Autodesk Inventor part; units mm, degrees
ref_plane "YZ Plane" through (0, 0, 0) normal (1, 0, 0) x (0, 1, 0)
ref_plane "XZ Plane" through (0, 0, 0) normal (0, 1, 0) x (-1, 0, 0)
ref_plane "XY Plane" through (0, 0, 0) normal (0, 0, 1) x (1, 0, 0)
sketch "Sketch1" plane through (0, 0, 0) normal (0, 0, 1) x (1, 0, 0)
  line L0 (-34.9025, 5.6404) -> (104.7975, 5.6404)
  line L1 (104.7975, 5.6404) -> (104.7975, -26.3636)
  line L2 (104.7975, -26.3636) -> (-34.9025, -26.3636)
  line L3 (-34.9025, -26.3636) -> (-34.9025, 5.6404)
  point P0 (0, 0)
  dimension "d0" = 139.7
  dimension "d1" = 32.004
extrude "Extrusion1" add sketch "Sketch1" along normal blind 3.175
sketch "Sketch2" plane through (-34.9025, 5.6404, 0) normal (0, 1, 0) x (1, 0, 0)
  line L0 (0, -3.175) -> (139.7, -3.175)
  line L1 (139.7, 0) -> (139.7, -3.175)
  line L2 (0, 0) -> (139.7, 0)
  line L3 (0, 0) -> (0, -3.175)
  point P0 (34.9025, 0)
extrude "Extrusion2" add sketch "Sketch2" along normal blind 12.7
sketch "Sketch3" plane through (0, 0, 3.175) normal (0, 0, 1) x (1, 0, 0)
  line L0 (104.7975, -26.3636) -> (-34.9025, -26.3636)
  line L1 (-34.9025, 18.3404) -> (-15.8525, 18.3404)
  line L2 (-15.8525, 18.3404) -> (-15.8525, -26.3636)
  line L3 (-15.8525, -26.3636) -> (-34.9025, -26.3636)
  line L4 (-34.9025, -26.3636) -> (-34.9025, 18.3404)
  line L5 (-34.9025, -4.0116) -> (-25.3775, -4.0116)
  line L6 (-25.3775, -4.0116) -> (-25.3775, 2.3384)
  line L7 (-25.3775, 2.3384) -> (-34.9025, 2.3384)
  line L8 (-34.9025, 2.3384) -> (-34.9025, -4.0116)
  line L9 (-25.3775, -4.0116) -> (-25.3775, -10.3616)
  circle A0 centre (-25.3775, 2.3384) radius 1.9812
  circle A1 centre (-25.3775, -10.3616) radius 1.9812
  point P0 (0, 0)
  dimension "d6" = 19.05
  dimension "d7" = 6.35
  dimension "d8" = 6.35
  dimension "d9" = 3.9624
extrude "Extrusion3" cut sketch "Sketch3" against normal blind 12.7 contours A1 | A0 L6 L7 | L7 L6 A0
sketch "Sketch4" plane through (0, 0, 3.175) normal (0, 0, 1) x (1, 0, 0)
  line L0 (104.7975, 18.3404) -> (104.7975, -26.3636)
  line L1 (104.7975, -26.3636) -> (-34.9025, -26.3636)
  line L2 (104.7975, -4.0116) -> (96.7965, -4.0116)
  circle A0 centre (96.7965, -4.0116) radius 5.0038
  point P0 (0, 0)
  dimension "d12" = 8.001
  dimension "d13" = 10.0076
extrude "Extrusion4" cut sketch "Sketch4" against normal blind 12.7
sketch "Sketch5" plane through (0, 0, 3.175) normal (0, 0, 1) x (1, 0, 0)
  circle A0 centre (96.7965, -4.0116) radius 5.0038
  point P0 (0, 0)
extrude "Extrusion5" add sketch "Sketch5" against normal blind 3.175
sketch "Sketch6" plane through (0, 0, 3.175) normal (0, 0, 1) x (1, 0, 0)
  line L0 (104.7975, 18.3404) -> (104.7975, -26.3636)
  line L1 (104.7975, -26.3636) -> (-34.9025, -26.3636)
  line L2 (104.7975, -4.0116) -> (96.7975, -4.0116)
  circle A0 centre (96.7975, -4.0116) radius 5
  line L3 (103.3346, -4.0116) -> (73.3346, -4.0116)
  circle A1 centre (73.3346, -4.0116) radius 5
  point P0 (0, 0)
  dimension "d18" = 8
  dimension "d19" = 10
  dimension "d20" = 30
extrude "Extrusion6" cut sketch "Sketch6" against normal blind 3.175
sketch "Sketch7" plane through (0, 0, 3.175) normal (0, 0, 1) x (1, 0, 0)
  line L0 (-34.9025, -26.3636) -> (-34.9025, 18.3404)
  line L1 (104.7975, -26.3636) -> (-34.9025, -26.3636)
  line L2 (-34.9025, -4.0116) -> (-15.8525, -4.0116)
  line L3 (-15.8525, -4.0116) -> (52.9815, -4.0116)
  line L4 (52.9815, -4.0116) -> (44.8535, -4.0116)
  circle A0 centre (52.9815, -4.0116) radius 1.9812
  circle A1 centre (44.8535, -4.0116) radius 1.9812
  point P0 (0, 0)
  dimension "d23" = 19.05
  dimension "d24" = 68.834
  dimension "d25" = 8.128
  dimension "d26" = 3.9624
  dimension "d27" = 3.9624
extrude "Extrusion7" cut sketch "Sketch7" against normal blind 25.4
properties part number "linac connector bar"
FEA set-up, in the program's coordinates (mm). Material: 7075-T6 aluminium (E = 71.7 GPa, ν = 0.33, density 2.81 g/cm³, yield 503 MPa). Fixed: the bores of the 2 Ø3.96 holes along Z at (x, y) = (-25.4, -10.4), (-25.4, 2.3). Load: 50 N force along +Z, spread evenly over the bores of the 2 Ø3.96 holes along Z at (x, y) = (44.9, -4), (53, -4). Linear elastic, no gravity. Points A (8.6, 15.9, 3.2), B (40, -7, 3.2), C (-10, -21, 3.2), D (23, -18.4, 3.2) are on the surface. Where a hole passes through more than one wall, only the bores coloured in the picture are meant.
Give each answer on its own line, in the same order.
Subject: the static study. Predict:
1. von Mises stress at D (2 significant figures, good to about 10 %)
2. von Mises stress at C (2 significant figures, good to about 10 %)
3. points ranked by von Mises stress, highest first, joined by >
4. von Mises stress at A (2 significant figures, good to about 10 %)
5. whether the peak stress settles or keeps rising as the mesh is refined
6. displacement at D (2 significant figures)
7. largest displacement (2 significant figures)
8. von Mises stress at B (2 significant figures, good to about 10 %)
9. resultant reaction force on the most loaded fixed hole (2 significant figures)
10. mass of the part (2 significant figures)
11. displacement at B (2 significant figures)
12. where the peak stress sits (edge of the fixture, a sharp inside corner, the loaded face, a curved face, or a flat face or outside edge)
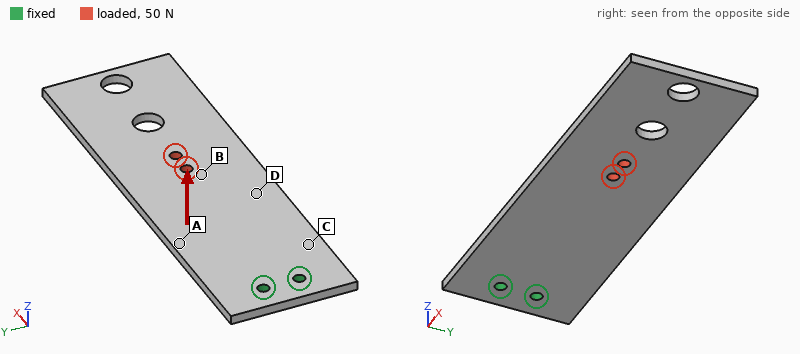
17 MPa
38 MPa
C > A > D > B
27 MPa
keeps rising
0.40 mm
1.7 mm
8.2 MPa
25 N
54 g
0.65 mm
edge of the fixture
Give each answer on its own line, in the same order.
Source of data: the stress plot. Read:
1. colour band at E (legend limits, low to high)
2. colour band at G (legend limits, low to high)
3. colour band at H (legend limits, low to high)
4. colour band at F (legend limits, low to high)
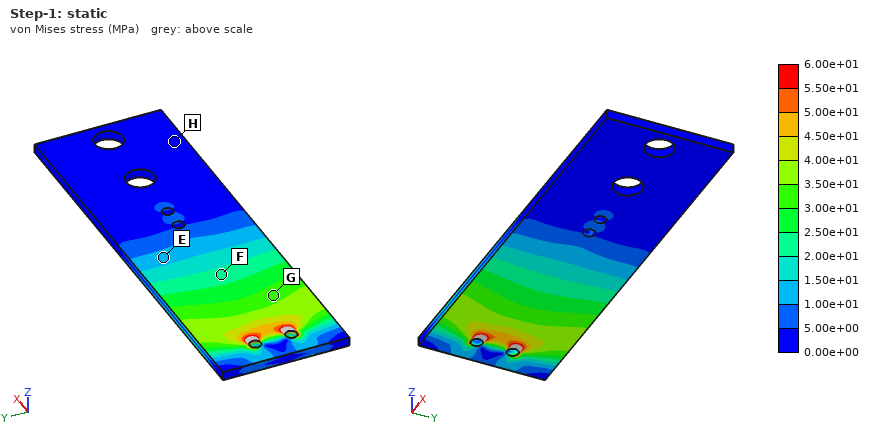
1.00e+01 to 1.50e+01 MPa
3.00e+01 to 3.50e+01 MPa
0.00e+00 to 5.00e+00 MPa
2.00e+01 to 2.50e+01 MPa
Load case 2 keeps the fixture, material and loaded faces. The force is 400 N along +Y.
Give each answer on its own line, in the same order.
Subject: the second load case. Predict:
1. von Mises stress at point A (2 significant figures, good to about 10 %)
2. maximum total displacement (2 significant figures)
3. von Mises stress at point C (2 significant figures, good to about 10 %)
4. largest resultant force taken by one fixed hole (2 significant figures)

14 MPa
0.17 mm
16 MPa
1.9 kN
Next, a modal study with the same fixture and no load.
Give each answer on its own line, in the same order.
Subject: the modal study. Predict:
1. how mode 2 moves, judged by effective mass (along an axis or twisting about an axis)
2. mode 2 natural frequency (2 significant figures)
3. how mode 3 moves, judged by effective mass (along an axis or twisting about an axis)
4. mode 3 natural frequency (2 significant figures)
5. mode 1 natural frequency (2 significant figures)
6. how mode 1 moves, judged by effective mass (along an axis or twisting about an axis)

twisting about X
860 Hz
along Z
960 Hz
160 Hz
along Z
